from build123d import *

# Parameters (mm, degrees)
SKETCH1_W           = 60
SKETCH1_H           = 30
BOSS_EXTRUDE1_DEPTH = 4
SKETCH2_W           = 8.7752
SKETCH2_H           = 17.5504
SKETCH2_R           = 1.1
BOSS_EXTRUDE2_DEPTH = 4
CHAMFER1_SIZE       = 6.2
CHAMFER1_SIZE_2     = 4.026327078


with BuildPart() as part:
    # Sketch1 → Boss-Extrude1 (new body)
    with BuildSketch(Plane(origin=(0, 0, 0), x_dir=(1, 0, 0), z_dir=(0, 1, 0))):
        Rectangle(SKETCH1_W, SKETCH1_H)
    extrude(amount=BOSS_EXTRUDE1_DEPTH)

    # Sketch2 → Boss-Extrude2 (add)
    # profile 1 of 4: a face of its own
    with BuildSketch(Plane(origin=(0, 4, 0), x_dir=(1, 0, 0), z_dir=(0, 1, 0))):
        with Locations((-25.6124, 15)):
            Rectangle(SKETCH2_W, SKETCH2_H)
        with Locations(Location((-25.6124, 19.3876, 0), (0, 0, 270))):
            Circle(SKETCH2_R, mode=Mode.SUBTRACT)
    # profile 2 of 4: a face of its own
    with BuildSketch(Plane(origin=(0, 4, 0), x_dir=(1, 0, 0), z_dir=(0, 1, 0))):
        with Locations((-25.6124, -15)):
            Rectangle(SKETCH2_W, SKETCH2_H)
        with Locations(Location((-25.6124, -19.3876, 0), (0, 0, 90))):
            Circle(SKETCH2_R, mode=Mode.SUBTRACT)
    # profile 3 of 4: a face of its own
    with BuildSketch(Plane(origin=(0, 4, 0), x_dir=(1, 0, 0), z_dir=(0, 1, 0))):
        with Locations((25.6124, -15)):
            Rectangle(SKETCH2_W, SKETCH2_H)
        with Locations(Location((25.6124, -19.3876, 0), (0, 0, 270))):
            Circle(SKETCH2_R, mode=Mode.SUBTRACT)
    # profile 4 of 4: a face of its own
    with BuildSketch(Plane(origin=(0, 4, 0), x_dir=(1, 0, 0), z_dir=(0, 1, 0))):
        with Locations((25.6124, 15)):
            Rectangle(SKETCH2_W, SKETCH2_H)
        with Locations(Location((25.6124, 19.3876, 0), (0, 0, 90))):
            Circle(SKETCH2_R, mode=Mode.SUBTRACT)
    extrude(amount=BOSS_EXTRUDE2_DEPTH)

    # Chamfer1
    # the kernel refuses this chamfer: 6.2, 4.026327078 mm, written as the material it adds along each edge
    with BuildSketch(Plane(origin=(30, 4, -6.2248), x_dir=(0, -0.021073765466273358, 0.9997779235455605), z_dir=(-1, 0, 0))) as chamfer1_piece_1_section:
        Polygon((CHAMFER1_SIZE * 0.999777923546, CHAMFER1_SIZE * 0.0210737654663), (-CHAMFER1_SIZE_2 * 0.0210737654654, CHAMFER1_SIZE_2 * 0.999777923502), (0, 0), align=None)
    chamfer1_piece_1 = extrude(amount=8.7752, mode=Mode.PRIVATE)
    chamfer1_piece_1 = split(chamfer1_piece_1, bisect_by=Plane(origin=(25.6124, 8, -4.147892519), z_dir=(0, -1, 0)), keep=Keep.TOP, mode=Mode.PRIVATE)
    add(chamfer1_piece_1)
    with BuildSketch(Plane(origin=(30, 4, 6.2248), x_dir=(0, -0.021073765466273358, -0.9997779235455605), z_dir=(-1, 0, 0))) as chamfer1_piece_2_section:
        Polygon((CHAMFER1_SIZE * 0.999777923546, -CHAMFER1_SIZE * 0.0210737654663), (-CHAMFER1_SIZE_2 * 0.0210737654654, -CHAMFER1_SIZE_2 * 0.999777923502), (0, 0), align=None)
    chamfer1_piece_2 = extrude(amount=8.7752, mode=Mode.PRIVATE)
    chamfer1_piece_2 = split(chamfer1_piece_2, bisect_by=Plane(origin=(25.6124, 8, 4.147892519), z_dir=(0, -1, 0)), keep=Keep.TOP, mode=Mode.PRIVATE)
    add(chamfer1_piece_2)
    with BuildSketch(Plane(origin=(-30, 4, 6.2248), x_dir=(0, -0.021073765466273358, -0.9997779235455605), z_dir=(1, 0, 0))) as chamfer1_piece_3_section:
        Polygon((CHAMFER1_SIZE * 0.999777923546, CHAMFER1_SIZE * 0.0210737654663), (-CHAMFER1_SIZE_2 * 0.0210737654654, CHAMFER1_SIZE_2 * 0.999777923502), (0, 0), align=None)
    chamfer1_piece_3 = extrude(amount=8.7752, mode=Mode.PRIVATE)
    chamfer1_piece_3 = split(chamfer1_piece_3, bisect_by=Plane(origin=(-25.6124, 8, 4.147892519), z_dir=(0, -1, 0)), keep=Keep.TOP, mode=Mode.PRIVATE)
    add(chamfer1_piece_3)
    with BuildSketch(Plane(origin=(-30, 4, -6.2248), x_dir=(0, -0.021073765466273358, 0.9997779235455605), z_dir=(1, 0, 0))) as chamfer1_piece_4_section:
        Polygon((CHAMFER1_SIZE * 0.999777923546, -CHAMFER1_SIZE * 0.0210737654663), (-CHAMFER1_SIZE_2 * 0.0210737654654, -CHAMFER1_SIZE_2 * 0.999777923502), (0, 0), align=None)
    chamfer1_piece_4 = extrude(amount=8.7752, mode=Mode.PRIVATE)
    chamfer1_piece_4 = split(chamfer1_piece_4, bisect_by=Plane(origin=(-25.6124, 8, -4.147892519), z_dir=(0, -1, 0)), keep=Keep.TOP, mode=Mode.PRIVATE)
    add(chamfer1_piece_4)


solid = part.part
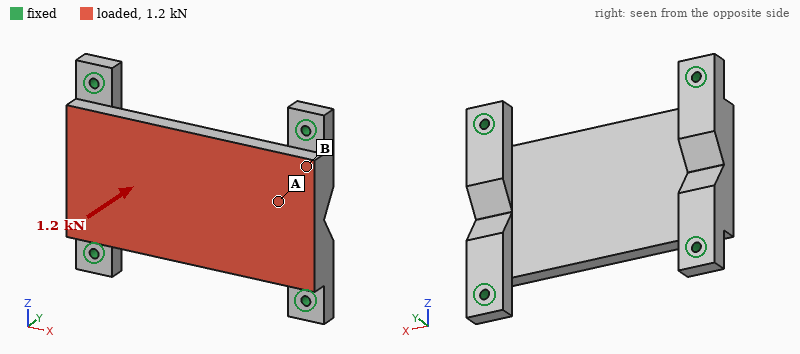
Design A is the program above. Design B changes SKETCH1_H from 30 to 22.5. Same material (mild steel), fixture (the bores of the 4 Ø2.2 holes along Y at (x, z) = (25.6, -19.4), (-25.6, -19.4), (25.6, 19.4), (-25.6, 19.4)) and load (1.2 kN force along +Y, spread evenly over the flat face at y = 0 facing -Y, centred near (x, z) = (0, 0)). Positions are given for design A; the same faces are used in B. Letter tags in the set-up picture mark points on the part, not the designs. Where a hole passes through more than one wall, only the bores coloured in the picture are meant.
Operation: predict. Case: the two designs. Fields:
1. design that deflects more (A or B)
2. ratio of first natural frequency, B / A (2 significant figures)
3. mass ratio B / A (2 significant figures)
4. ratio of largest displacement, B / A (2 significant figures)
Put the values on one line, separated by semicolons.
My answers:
B; 0.93; 0.82; 1.6
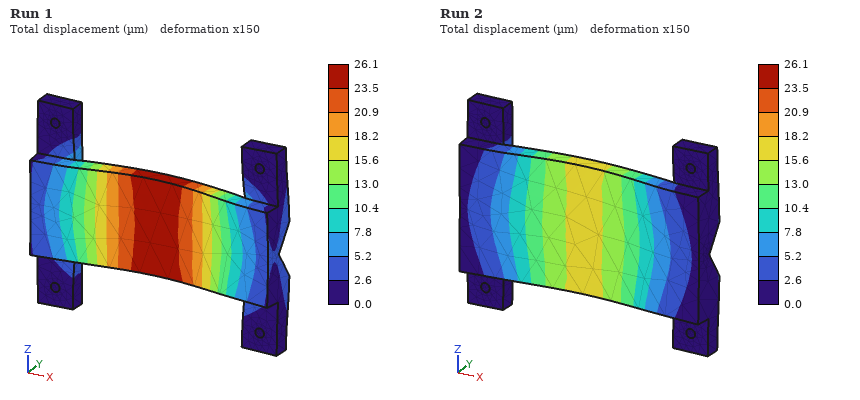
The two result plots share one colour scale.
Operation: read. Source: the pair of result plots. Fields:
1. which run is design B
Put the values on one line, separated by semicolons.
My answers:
Run 1
